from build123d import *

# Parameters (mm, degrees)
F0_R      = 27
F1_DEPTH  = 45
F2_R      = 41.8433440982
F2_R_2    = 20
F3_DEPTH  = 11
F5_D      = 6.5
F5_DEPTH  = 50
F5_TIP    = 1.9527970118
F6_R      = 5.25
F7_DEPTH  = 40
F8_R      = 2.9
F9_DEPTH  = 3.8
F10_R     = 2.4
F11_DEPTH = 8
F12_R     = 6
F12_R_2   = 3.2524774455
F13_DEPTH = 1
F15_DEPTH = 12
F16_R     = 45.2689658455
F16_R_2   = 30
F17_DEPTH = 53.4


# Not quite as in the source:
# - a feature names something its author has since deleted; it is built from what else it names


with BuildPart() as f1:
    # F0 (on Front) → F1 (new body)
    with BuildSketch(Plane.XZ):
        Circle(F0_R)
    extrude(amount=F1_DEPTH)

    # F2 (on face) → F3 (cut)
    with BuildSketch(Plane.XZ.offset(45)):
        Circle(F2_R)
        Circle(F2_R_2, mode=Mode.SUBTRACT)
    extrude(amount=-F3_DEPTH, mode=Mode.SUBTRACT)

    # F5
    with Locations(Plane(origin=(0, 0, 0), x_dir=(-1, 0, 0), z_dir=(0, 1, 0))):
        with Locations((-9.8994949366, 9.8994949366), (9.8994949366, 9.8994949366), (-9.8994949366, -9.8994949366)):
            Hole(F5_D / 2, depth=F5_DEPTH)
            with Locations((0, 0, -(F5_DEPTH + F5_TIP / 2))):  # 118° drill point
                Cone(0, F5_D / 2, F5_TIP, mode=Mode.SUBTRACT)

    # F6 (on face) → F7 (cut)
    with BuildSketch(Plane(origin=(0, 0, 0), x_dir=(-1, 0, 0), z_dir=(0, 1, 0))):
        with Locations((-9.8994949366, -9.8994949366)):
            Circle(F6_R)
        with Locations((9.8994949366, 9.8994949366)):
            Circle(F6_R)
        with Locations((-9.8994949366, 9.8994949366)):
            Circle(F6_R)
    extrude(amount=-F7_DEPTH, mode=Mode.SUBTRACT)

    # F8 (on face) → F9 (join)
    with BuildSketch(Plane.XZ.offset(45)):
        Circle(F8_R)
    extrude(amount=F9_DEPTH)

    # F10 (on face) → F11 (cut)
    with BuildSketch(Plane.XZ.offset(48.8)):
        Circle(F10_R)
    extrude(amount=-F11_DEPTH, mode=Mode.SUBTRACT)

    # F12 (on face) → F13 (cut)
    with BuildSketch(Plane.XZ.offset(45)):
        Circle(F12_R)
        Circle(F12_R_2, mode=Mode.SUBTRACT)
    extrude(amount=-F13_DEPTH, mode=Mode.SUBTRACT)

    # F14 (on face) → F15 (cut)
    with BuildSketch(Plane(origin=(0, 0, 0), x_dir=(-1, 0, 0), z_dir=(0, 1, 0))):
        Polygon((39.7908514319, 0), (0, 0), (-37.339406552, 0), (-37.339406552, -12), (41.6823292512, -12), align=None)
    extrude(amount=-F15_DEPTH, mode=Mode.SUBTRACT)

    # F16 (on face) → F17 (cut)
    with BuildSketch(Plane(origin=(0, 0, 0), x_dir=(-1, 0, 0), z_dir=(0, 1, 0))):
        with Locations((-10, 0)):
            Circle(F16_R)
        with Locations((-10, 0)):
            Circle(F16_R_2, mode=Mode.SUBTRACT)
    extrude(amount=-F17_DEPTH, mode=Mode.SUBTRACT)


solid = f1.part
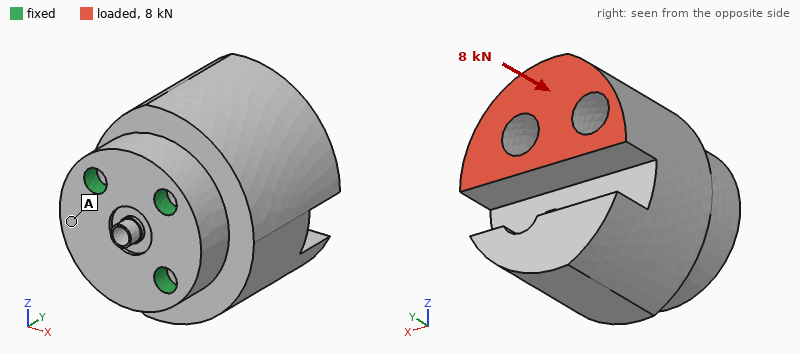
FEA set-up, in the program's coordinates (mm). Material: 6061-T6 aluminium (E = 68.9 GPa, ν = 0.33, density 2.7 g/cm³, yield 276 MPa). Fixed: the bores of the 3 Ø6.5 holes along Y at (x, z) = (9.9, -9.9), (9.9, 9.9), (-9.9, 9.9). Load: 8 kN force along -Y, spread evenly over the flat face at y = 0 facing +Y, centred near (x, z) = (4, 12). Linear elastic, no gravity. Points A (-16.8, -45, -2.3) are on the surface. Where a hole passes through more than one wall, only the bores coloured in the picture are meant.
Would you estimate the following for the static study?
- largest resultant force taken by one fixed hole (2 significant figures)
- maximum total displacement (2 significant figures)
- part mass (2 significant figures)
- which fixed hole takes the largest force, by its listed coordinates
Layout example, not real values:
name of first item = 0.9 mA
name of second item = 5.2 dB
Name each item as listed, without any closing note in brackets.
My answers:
largest resultant force taken by one fixed hole = 5.2 kN
maximum total displacement = 40 µm
part mass = 170 g
which fixed hole takes the largest force, by its listed coordinates = (9.9, 9.9)
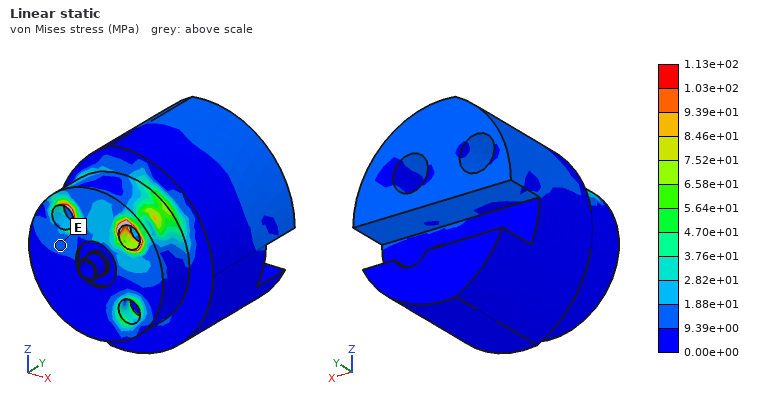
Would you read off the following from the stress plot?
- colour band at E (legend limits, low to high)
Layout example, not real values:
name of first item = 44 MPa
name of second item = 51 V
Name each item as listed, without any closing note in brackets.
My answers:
colour band at E = 9.39e+00 to 1.88e+01 MPa
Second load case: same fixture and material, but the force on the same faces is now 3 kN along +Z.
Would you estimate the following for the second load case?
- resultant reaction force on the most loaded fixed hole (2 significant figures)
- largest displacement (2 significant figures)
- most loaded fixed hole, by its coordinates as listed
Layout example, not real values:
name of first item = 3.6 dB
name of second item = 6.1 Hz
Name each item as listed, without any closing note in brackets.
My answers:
resultant reaction force on the most loaded fixed hole = 5.3 kN
largest displacement = 67 µm
most loaded fixed hole, by its coordinates as listed = (9.9, -9.9)
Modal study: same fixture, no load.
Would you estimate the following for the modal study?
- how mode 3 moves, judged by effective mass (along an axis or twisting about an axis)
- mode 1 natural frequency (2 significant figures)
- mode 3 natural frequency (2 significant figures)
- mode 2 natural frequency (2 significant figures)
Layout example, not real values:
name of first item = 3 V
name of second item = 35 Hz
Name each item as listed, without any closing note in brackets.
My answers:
how mode 3 moves, judged by effective mass = twisting about Y
mode 1 natural frequency = 4000 Hz
mode 3 natural frequency = 10 kHz
mode 2 natural frequency = 6000 Hz
